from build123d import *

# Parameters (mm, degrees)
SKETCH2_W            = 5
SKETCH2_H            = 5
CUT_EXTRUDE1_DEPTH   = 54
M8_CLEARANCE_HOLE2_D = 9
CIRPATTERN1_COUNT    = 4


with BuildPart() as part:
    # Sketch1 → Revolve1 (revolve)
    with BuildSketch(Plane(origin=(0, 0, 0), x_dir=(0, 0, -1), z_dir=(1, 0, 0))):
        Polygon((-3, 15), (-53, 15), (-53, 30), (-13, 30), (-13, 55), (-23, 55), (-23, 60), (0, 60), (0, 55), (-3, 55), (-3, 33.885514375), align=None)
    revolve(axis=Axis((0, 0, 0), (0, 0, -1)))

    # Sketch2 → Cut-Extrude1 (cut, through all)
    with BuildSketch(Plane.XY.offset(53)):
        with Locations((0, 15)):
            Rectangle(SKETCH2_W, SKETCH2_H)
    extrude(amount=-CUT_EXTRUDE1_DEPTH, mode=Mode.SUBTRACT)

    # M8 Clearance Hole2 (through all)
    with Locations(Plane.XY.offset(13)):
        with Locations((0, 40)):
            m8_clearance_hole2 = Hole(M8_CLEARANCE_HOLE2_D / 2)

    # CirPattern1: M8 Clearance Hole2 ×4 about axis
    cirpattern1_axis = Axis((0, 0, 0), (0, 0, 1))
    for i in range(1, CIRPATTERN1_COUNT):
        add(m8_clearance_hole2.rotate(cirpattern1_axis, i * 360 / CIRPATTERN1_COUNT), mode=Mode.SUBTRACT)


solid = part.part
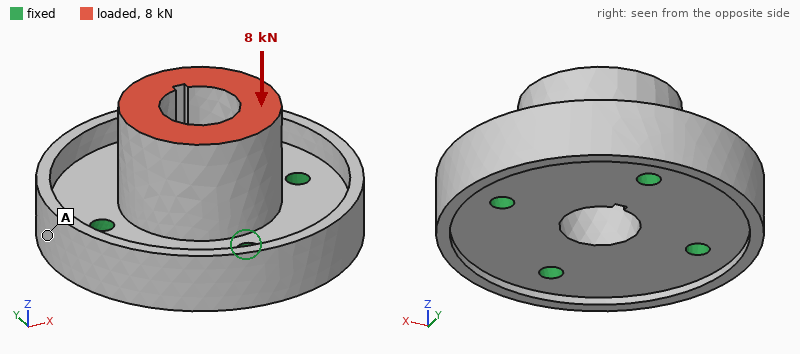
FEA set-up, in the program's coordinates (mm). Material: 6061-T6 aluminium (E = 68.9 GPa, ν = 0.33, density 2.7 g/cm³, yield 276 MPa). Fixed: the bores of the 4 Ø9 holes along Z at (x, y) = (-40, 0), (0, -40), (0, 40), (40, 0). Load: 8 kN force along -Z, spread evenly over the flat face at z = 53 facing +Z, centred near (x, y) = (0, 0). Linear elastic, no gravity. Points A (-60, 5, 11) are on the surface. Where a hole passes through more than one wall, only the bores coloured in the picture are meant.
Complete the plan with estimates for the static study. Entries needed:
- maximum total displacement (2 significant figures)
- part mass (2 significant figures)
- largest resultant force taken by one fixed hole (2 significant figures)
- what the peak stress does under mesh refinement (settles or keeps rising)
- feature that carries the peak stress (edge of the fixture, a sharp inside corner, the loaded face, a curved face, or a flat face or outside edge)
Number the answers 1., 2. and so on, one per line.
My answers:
1. 8.3 µm
2. 570 g
3. 2.1 kN
4. keeps rising
5. edge of the fixture
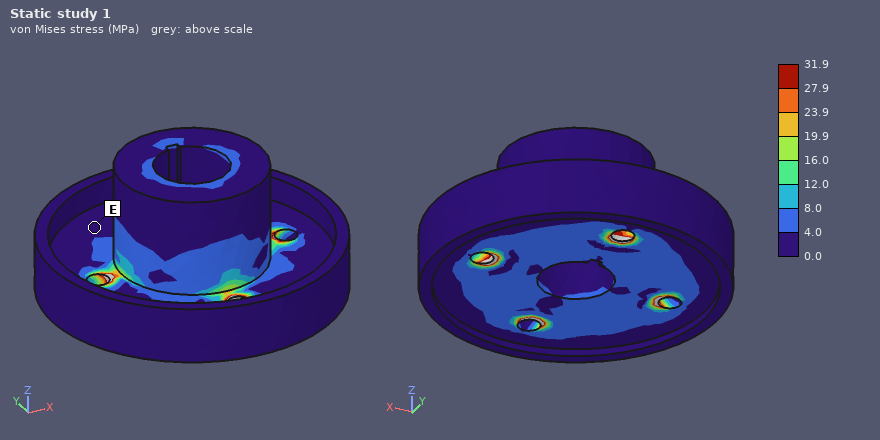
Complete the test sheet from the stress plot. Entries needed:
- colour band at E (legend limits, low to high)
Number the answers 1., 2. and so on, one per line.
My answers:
1. 0.0 to 4.0 MPa
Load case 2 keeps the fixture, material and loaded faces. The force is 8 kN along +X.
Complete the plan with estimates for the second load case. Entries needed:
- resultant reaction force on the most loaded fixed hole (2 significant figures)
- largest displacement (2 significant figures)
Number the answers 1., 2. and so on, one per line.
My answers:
1. 5.5 kN
2. 40 µm
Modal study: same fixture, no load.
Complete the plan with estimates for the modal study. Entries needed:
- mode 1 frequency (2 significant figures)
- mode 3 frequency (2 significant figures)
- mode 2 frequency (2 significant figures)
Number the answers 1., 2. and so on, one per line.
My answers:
1. 6700 Hz
2. 7300 Hz
3. 7300 Hz
